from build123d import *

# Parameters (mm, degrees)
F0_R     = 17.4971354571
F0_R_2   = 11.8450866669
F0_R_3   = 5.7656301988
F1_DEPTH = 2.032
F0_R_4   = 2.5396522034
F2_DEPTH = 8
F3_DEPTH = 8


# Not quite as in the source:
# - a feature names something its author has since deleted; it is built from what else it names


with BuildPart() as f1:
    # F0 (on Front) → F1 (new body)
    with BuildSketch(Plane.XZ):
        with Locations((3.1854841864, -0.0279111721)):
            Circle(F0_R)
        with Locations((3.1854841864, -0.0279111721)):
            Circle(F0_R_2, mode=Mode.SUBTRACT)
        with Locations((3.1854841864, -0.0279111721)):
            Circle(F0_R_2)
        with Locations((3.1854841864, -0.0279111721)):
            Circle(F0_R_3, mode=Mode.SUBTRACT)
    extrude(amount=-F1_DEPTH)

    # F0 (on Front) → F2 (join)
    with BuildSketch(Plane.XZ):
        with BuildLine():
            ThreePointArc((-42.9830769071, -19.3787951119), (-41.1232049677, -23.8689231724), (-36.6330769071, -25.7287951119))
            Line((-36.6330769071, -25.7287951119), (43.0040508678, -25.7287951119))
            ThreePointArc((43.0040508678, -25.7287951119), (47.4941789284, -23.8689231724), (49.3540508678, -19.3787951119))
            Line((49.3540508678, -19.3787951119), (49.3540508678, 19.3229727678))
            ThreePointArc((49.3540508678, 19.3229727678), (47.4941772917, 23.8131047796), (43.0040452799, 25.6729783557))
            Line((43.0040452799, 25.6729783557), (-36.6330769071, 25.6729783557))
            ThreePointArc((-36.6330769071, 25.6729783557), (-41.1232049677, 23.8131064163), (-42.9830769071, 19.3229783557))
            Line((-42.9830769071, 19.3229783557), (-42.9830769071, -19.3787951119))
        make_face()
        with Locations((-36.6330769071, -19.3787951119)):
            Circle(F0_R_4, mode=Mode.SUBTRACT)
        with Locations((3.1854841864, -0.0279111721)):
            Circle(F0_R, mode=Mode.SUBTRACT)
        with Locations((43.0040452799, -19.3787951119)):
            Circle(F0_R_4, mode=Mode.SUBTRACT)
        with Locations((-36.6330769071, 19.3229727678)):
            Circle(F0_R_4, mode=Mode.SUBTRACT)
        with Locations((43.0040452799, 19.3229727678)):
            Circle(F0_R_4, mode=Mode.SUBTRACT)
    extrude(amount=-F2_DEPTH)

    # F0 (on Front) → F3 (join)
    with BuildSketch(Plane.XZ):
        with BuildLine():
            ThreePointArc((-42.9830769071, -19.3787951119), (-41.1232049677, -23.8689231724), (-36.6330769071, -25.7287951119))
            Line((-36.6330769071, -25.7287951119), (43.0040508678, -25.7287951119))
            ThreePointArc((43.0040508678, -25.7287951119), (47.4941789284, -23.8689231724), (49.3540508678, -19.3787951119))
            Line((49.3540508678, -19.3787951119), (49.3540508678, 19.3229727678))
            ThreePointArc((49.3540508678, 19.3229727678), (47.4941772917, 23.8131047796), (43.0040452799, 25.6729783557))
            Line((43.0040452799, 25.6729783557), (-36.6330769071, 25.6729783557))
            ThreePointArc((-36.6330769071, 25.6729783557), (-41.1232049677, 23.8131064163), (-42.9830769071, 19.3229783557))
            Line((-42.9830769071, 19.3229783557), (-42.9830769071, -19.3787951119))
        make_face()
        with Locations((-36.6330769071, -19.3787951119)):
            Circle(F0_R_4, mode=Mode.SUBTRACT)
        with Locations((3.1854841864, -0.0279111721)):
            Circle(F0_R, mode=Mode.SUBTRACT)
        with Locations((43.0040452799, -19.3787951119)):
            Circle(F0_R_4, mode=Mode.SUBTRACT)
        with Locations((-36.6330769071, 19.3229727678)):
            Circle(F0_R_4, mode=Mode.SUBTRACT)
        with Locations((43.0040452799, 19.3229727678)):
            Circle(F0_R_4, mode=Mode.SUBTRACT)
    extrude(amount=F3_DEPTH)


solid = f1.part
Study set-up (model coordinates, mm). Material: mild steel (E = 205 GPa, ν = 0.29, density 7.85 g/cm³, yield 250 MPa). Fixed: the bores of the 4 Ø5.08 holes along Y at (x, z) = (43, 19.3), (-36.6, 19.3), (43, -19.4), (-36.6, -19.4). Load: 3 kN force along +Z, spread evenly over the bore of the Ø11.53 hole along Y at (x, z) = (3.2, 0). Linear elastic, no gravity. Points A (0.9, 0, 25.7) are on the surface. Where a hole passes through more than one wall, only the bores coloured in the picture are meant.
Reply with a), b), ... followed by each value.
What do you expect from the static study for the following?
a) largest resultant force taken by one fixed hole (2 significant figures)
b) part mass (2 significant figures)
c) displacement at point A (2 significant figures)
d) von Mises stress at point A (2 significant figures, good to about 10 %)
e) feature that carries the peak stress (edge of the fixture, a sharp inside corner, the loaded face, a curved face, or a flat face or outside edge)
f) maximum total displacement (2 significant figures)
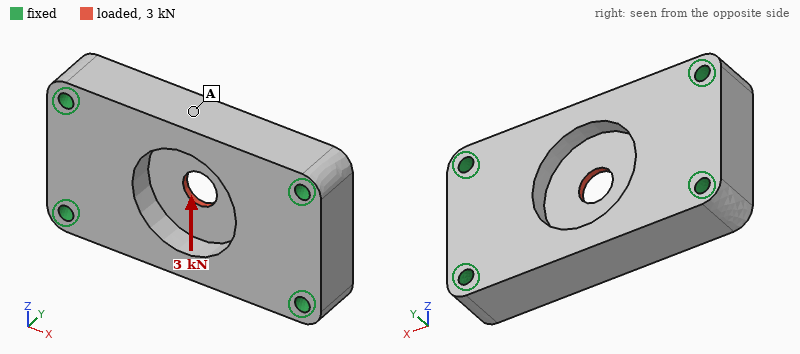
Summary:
a) 1.0 kN
b) 470 g
c) 1.5 µm
d) 8.5 MPa
e) the loaded face
f) 3.4 µm
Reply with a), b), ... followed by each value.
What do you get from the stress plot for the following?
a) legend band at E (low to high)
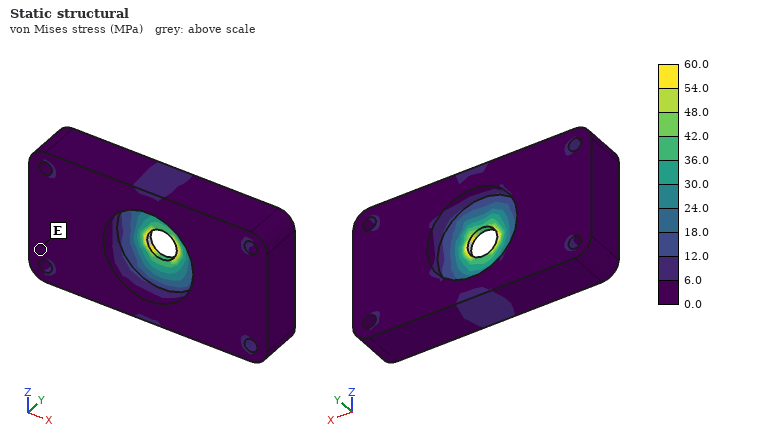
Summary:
a) 0.0 to 6.0 MPa
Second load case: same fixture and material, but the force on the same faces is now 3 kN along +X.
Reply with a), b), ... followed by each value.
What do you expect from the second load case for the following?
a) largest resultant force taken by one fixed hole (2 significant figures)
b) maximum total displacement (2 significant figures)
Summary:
a) 780 N
b) 2.5 µm
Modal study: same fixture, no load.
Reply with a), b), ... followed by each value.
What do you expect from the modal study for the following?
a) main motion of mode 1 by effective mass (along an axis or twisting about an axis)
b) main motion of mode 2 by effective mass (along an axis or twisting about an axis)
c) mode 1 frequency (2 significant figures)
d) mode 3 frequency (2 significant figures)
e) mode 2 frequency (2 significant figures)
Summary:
a) along Y
b) twisting about X
c) 10 kHz
d) 18 kHz
e) 14 kHz
